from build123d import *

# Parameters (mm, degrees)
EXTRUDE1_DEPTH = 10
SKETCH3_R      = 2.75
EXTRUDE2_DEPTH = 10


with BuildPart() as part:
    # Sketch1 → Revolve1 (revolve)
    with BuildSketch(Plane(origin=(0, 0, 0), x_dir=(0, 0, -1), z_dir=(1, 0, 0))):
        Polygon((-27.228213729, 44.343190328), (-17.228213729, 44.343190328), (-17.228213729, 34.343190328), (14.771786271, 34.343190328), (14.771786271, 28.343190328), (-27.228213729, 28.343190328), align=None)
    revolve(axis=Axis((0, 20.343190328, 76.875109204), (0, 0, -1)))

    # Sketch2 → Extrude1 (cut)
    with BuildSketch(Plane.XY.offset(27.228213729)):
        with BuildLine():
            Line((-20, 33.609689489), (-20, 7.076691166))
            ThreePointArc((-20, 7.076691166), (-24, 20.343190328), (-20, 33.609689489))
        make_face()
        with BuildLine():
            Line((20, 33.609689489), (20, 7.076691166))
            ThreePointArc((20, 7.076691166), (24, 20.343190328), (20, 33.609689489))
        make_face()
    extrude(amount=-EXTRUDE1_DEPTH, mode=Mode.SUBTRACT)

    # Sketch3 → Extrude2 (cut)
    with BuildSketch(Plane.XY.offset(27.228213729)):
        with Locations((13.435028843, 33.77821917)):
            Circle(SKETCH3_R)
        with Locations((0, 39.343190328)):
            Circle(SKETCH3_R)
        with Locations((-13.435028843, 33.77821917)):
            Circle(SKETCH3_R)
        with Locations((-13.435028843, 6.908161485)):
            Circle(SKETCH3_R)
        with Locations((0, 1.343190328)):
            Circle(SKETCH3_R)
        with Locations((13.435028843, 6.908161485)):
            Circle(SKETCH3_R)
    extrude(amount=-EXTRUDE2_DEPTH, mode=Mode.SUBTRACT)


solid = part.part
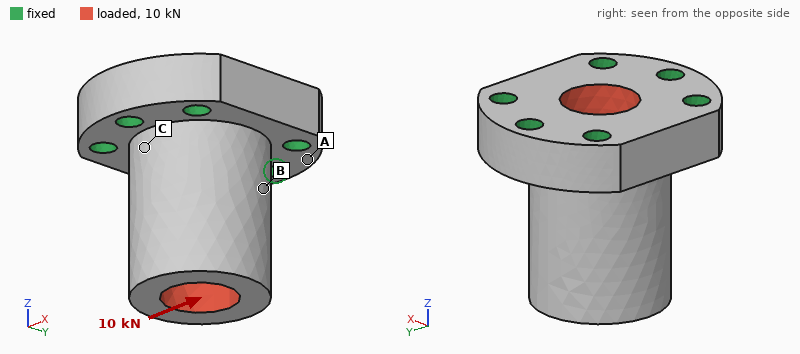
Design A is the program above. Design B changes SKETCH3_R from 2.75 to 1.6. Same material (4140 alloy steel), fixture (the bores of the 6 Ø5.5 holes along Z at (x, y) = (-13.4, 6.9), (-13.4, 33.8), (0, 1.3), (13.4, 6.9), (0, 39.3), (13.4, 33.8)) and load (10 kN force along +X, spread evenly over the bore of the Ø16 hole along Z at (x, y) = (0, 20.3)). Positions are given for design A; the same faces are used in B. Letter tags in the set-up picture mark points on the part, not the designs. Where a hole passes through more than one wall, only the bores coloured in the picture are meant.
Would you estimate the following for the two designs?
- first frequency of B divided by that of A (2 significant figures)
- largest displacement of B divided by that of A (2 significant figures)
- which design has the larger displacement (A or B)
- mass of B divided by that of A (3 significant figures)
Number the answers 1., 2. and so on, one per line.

1. 0.94
2. 1.1
3. B
4. 1.04
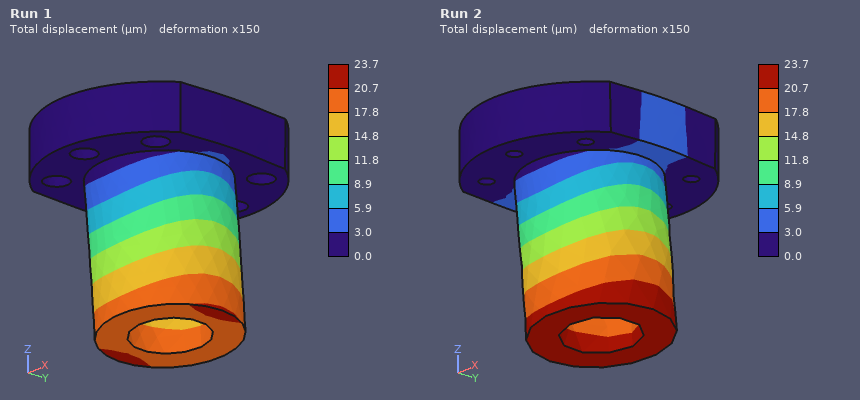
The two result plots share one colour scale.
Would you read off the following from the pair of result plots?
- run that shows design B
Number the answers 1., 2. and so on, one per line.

1. Run 2
